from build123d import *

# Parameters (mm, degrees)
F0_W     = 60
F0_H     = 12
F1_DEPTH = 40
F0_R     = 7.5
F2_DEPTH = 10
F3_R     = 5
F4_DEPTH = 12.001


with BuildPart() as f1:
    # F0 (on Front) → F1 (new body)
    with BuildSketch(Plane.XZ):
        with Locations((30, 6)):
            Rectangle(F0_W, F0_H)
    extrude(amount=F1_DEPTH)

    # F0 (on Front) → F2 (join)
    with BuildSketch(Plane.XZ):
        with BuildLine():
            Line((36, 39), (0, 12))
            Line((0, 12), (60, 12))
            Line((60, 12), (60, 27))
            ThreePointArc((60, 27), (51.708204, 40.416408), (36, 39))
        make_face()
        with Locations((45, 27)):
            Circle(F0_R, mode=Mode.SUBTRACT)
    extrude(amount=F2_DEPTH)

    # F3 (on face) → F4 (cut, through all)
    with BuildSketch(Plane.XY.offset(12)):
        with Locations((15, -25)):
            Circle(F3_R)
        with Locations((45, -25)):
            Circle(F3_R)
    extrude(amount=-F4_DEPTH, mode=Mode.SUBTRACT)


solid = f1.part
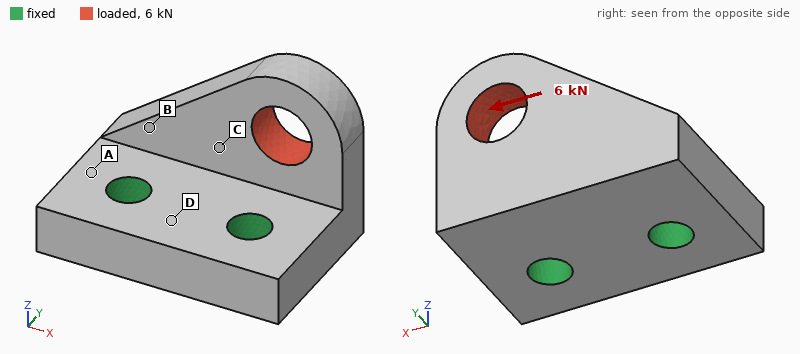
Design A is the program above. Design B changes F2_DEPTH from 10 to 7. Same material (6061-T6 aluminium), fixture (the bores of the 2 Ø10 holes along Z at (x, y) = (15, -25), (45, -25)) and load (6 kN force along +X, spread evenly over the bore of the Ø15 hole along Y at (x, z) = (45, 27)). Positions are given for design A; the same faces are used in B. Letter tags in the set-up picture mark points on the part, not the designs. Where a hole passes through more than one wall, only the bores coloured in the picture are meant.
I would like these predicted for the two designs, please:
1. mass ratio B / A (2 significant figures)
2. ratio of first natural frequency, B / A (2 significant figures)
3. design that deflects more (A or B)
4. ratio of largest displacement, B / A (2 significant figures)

0.92
0.92
B
1.3
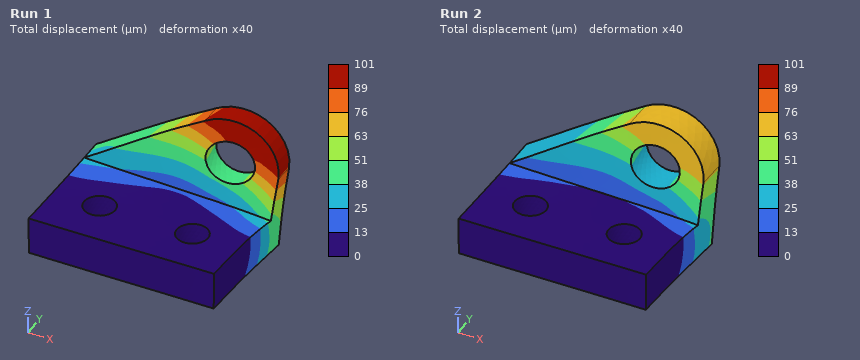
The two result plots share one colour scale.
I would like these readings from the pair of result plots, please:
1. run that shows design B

Run 1
